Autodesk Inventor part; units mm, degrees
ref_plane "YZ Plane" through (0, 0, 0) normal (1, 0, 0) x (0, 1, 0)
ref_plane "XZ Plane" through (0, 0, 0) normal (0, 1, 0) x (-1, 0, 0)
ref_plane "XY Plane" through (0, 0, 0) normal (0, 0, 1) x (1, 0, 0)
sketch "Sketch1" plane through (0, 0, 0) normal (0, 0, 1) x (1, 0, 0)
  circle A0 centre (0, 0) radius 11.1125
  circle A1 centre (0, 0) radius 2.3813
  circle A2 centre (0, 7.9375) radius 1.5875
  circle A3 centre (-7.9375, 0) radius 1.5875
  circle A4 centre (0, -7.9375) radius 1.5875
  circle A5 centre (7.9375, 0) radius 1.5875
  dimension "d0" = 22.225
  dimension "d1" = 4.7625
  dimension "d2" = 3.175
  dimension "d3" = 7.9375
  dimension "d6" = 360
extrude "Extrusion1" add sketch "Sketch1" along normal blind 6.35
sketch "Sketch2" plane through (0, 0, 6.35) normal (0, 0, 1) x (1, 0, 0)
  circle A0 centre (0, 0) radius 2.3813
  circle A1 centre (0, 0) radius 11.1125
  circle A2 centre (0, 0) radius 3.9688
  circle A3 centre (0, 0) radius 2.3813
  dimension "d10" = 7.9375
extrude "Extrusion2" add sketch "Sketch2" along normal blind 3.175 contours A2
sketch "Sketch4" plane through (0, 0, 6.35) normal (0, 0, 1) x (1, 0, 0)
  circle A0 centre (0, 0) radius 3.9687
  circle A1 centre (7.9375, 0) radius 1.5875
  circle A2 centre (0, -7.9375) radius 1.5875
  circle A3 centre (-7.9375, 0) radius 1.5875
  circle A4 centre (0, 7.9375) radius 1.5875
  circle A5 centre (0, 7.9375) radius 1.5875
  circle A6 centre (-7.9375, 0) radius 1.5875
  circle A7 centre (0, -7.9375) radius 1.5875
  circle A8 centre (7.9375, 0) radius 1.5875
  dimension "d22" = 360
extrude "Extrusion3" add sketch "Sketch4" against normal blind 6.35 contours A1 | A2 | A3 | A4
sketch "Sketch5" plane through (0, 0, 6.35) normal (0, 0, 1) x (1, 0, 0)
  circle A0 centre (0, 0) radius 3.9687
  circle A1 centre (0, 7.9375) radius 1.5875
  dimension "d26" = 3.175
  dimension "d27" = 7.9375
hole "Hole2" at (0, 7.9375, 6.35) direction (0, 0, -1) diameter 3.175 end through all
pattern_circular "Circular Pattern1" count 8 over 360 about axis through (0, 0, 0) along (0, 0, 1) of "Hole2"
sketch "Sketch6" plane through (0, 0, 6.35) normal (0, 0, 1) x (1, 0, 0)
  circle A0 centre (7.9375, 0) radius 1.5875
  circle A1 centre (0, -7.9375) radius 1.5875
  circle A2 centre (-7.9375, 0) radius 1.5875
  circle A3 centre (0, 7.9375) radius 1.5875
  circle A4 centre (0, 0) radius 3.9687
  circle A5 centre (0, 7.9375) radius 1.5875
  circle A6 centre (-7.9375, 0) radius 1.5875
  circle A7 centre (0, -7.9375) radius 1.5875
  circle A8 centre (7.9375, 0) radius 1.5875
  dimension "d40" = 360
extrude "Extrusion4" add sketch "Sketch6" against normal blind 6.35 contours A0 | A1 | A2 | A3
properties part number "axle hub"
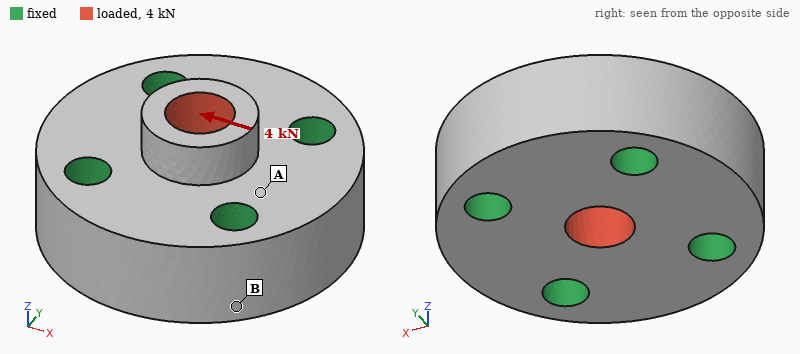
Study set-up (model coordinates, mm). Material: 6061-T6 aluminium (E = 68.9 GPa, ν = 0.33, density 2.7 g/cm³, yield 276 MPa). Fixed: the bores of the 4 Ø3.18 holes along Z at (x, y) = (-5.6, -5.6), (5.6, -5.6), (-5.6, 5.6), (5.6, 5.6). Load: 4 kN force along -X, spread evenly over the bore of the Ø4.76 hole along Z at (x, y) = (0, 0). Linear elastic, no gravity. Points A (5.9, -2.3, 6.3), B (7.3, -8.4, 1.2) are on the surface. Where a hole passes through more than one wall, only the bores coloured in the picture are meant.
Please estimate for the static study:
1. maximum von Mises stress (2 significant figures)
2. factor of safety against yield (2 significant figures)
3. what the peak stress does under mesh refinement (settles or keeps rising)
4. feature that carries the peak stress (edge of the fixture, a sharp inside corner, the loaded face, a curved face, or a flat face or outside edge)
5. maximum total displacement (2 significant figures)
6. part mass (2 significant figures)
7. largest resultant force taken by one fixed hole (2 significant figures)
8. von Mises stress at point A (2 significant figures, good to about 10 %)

120 MPa
2.3
settles
the loaded face
12 µm
6.1 g
1.1 kN
25 MPa
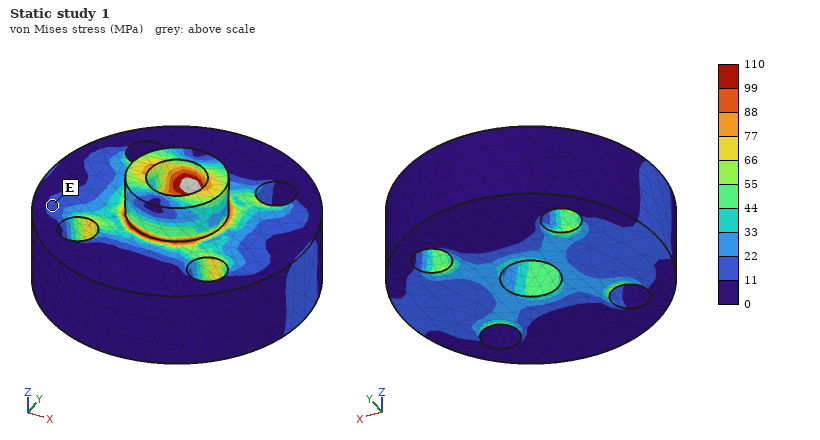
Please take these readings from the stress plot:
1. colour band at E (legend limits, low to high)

11 to 22 MPa
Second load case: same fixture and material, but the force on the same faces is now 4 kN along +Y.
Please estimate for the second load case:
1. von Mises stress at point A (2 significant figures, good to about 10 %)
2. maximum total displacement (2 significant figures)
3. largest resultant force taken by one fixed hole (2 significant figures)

15 MPa
12 µm
1.1 kN
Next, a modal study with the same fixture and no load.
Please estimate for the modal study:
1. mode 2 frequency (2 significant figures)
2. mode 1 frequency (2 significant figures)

110 kHz
110 kHz
